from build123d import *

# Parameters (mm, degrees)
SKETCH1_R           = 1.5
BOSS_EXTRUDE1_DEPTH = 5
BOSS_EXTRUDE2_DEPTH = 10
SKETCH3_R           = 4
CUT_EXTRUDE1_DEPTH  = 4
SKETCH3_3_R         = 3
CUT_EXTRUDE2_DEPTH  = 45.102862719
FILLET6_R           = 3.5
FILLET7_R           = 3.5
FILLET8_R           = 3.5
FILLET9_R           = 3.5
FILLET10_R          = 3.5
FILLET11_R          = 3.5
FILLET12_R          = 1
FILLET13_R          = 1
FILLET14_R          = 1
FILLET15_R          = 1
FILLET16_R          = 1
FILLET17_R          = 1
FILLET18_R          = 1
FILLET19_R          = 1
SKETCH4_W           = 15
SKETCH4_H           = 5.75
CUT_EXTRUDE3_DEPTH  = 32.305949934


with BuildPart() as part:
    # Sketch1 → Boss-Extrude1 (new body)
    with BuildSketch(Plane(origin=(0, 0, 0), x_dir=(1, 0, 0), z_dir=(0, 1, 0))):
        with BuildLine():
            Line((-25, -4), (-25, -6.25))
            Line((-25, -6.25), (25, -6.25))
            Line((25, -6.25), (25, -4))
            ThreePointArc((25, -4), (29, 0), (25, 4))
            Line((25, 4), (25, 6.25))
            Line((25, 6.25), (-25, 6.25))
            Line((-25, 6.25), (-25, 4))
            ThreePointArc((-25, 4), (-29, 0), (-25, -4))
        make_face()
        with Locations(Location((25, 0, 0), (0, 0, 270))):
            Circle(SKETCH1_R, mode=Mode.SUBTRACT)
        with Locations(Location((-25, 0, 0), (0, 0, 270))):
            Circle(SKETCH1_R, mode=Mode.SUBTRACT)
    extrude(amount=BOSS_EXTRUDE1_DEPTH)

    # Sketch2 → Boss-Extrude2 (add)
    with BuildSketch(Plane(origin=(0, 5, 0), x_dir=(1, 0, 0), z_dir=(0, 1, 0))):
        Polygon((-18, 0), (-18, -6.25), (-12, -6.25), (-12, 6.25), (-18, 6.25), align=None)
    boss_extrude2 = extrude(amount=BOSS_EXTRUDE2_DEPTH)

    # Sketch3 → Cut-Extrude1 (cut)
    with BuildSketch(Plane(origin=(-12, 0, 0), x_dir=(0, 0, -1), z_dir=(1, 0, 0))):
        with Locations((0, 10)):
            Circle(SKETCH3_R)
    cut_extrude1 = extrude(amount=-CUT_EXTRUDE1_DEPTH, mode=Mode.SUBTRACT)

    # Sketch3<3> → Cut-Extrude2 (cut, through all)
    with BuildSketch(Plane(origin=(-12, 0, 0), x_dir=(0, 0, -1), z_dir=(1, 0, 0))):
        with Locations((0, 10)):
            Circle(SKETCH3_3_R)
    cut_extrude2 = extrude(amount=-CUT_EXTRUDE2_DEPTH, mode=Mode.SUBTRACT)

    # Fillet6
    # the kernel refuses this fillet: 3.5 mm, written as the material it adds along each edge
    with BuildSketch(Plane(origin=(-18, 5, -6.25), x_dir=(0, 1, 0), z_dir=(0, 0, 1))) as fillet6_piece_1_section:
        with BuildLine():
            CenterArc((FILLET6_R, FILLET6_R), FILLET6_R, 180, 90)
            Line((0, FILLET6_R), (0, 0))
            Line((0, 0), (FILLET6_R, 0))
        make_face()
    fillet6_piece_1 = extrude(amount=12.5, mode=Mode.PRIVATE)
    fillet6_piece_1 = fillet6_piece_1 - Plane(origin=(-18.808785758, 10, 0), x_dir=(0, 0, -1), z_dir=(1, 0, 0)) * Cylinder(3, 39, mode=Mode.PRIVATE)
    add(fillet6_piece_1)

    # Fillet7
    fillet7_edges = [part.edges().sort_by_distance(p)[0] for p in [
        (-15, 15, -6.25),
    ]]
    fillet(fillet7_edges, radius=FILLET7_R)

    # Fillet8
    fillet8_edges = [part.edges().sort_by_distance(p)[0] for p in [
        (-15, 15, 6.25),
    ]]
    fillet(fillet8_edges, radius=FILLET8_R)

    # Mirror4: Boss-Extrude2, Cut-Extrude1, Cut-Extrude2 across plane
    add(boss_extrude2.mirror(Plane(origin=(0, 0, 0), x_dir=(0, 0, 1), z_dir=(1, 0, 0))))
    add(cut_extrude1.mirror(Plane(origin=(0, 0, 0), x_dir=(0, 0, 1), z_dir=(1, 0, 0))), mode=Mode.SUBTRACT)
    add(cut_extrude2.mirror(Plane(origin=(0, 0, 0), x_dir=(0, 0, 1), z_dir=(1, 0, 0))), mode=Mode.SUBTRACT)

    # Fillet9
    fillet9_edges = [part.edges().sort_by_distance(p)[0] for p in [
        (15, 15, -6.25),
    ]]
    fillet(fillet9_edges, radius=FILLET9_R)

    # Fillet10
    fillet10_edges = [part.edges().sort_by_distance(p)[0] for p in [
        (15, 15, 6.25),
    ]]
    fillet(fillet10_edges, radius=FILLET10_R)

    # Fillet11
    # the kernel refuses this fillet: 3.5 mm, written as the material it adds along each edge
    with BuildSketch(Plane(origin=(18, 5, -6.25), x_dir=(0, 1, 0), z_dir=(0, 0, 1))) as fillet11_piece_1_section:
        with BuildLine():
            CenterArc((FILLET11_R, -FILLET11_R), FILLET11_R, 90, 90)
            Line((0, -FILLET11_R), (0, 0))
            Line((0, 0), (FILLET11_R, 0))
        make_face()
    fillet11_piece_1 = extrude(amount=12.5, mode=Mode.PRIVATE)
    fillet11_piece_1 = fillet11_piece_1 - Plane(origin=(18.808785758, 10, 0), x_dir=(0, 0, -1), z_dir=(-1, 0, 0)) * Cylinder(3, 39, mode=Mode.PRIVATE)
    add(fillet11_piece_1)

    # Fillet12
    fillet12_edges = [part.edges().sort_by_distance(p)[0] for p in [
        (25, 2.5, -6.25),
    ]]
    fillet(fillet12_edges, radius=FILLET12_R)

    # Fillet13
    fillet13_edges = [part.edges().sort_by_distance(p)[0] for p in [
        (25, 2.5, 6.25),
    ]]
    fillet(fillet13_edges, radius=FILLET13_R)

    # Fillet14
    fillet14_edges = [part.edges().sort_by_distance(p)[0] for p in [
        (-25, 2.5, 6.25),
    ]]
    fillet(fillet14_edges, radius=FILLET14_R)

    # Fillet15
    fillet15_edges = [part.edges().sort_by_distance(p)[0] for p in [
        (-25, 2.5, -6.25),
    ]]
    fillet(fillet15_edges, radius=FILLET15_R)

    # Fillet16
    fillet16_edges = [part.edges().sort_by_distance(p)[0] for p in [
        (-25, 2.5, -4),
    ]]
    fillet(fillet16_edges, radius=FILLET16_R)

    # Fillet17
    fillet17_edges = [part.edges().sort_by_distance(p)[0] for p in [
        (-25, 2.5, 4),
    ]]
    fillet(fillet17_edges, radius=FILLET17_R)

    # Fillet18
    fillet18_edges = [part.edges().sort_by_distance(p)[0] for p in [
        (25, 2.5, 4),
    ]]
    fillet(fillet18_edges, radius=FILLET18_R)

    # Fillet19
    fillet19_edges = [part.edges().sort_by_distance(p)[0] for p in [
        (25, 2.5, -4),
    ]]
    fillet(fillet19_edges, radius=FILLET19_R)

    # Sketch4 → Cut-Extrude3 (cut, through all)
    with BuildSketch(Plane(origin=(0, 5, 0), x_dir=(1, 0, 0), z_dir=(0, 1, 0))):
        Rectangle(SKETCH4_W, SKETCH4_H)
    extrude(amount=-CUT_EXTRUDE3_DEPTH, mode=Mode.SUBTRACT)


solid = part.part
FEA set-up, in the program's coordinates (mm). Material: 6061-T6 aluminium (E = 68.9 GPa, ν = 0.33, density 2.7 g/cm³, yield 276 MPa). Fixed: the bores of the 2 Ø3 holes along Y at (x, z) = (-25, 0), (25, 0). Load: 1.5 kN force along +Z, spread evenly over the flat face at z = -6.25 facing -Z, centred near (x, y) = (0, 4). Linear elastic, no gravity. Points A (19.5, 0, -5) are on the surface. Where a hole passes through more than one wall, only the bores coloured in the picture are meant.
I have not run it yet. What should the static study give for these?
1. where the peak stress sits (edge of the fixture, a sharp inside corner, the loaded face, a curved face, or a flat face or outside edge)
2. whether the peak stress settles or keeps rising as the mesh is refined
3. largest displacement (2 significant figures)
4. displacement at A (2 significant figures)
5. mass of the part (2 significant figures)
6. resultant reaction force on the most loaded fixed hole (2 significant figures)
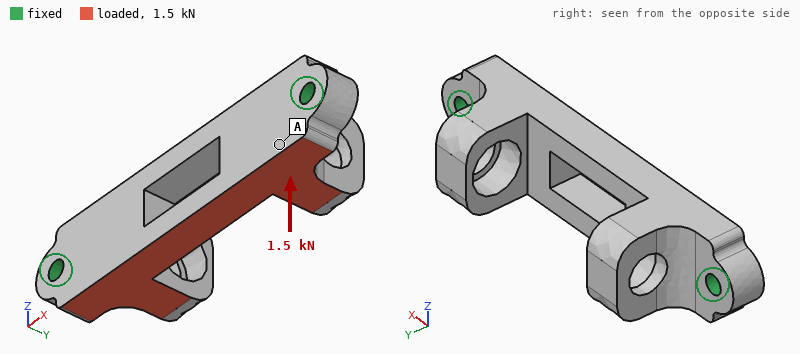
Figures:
edge of the fixture
keeps rising
36 µm
10.0 µm
10 g
750 N
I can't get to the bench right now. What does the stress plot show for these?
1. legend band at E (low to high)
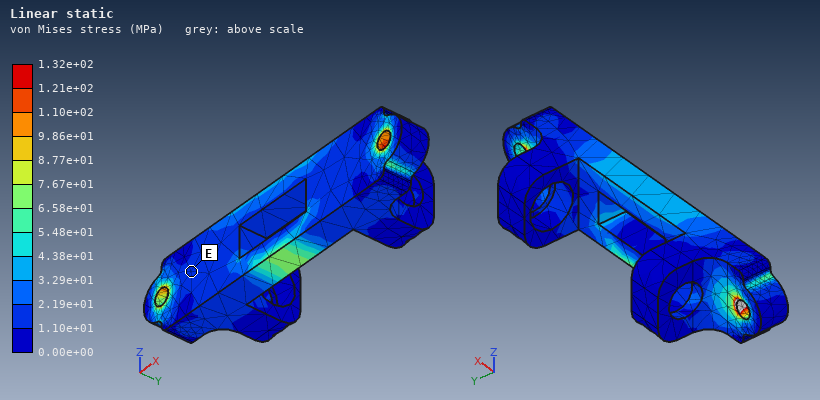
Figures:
1.10e+01 to 2.19e+01 MPa
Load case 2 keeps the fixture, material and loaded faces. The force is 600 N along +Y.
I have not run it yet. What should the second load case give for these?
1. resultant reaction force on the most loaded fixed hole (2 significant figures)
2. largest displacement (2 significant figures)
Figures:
300 N
44 µm
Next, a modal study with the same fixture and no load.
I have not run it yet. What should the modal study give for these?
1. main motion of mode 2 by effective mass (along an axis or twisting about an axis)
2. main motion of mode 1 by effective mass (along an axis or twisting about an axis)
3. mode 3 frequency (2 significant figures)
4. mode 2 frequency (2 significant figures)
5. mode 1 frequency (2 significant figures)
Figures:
along Z
along Y
15 kHz
13 kHz
8800 Hz
